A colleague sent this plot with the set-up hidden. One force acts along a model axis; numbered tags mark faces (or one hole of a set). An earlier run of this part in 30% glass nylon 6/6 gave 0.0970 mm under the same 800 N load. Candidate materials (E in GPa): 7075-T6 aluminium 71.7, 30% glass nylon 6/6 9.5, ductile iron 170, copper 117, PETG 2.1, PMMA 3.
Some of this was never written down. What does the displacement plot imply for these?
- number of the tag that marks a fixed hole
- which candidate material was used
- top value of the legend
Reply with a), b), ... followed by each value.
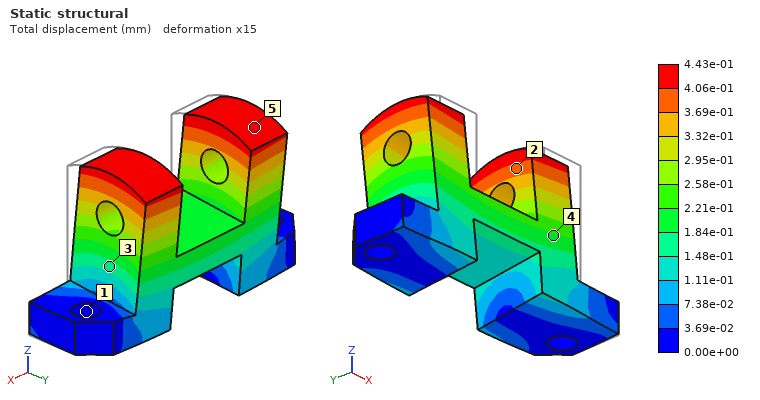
a) 1
b) PETG
c) 4.43e-01 mm
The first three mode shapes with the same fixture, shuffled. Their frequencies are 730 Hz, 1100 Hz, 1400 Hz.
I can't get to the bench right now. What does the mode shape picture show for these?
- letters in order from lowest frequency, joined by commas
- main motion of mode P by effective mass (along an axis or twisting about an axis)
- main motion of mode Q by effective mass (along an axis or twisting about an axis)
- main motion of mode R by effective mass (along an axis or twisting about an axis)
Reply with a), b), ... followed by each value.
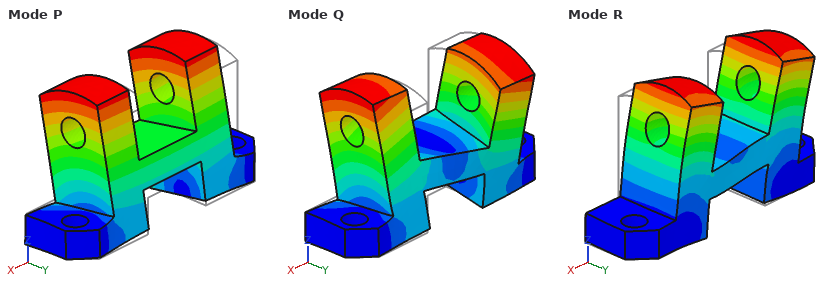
a) P, Q, R
b) along Y
c) twisting about Z
d) along X
